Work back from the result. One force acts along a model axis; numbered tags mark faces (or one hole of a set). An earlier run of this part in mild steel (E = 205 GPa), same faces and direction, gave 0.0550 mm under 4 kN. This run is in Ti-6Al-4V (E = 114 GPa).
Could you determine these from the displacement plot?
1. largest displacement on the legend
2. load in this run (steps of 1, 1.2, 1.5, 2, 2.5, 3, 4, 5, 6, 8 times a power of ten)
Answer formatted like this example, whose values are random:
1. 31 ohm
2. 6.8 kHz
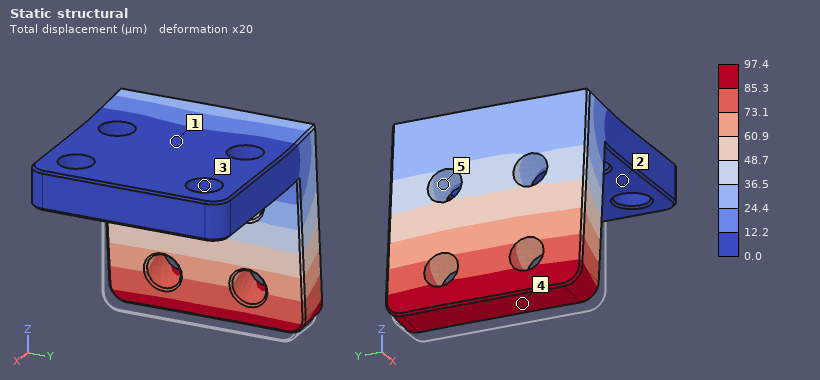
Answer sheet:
1. 97.4 µm
2. 4 kN
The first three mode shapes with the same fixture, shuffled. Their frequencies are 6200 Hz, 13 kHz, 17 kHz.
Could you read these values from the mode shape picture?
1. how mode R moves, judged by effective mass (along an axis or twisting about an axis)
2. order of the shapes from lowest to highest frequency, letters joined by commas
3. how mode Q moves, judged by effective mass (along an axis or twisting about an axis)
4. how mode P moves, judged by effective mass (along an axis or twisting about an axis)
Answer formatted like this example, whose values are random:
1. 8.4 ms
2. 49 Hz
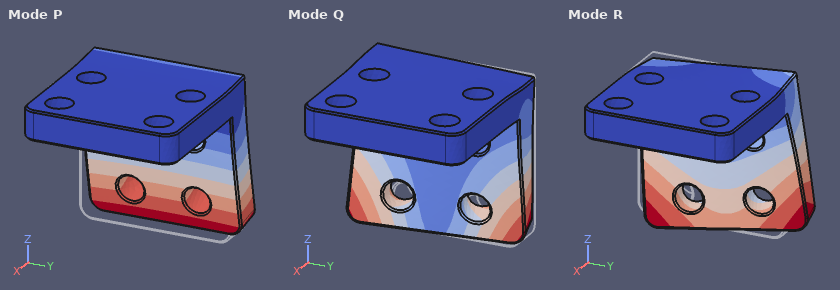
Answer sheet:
1. along Y
2. P, R, Q
3. along Y
4. along X
